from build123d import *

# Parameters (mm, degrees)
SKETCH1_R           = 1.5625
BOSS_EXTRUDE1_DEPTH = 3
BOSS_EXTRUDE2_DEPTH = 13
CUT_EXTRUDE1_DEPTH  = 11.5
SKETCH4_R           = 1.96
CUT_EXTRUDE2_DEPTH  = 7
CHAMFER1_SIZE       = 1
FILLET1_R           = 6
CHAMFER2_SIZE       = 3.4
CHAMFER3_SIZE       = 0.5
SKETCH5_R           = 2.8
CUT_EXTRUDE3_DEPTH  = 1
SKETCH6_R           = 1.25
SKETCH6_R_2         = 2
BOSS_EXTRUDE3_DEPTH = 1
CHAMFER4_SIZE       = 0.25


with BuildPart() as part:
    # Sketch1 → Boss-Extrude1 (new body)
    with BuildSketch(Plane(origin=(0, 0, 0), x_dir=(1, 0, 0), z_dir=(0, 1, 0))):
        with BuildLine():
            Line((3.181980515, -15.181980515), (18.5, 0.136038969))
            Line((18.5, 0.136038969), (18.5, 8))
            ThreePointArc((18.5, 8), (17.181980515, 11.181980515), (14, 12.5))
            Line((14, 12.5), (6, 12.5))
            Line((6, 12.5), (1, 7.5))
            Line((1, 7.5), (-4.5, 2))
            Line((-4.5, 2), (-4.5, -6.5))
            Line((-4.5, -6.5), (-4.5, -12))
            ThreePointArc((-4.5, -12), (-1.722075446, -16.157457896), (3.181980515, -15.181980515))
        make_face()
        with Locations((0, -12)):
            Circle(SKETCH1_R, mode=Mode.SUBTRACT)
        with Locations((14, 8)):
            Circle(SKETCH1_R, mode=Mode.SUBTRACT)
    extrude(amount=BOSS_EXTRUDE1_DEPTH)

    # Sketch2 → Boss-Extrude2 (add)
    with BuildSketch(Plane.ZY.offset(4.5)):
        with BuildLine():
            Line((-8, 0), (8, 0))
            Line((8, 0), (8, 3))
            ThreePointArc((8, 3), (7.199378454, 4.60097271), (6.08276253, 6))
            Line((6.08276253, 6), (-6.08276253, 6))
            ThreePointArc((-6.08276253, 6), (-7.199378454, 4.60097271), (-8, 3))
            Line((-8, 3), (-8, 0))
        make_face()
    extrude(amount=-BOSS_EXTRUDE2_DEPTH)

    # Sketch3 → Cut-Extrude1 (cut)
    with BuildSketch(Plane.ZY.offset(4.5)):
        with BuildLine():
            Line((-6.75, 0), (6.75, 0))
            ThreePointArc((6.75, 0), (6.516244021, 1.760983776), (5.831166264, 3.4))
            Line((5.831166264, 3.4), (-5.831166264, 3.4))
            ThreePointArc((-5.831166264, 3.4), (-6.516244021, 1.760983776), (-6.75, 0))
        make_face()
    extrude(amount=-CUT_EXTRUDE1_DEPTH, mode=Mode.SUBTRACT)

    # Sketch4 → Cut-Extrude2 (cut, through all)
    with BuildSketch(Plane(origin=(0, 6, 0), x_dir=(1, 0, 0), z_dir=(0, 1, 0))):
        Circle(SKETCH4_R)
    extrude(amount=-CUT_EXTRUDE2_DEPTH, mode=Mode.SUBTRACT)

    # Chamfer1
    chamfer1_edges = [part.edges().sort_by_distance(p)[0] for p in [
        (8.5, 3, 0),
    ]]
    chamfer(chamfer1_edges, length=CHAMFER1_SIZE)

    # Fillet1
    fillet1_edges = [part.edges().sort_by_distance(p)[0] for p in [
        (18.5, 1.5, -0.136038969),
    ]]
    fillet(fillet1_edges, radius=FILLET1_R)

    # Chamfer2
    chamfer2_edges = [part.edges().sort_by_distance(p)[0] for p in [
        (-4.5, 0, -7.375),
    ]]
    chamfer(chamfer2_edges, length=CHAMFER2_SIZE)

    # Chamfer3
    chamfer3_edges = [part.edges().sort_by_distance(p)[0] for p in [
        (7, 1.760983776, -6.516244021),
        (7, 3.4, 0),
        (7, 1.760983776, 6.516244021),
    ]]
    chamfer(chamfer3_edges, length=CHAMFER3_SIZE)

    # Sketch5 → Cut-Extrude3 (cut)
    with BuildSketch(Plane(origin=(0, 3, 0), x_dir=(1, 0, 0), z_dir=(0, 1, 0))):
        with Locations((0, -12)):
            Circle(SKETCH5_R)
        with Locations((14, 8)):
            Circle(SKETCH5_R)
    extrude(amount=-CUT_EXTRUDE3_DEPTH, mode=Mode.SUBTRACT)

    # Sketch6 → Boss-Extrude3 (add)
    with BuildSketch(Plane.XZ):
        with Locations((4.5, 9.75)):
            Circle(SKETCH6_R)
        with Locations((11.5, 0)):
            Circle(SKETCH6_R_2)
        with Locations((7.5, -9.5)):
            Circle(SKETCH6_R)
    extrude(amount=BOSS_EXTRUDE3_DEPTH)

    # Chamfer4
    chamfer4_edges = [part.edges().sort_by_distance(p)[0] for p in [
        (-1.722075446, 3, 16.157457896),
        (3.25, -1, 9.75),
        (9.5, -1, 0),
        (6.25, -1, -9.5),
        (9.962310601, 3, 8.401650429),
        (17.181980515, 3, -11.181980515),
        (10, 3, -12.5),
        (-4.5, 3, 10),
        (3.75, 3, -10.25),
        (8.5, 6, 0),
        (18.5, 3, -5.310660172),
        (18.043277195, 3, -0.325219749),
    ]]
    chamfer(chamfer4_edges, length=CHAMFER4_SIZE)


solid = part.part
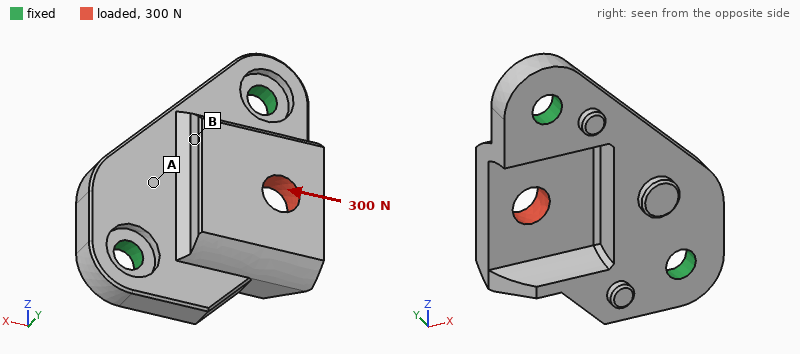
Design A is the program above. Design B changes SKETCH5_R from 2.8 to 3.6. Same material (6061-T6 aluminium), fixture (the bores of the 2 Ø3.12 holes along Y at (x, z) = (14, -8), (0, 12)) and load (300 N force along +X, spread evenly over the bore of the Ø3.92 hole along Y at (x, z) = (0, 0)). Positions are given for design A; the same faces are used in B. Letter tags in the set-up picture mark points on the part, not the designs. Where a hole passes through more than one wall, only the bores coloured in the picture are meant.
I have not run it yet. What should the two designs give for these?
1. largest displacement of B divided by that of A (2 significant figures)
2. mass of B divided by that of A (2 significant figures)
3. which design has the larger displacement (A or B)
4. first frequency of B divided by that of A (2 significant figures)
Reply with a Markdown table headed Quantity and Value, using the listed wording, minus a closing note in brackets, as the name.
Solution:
| Quantity | Value |
|---|---|
| largest displacement of B divided by that of A | 1.1 |
| mass of B divided by that of A | 0.98 |
| which design has the larger displacement | B |
| first frequency of B divided by that of A | 0.96 |
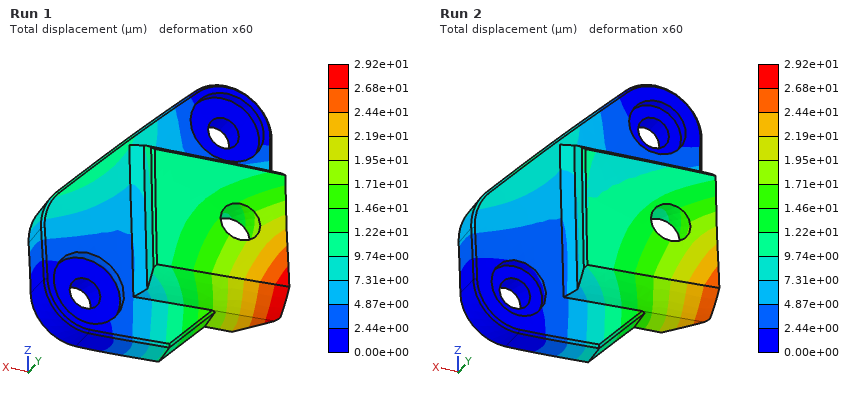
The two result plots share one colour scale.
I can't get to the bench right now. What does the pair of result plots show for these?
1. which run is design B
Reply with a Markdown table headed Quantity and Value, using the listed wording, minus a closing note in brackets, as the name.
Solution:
| Quantity | Value |
|---|---|
| which run is design B | Run 1 |
